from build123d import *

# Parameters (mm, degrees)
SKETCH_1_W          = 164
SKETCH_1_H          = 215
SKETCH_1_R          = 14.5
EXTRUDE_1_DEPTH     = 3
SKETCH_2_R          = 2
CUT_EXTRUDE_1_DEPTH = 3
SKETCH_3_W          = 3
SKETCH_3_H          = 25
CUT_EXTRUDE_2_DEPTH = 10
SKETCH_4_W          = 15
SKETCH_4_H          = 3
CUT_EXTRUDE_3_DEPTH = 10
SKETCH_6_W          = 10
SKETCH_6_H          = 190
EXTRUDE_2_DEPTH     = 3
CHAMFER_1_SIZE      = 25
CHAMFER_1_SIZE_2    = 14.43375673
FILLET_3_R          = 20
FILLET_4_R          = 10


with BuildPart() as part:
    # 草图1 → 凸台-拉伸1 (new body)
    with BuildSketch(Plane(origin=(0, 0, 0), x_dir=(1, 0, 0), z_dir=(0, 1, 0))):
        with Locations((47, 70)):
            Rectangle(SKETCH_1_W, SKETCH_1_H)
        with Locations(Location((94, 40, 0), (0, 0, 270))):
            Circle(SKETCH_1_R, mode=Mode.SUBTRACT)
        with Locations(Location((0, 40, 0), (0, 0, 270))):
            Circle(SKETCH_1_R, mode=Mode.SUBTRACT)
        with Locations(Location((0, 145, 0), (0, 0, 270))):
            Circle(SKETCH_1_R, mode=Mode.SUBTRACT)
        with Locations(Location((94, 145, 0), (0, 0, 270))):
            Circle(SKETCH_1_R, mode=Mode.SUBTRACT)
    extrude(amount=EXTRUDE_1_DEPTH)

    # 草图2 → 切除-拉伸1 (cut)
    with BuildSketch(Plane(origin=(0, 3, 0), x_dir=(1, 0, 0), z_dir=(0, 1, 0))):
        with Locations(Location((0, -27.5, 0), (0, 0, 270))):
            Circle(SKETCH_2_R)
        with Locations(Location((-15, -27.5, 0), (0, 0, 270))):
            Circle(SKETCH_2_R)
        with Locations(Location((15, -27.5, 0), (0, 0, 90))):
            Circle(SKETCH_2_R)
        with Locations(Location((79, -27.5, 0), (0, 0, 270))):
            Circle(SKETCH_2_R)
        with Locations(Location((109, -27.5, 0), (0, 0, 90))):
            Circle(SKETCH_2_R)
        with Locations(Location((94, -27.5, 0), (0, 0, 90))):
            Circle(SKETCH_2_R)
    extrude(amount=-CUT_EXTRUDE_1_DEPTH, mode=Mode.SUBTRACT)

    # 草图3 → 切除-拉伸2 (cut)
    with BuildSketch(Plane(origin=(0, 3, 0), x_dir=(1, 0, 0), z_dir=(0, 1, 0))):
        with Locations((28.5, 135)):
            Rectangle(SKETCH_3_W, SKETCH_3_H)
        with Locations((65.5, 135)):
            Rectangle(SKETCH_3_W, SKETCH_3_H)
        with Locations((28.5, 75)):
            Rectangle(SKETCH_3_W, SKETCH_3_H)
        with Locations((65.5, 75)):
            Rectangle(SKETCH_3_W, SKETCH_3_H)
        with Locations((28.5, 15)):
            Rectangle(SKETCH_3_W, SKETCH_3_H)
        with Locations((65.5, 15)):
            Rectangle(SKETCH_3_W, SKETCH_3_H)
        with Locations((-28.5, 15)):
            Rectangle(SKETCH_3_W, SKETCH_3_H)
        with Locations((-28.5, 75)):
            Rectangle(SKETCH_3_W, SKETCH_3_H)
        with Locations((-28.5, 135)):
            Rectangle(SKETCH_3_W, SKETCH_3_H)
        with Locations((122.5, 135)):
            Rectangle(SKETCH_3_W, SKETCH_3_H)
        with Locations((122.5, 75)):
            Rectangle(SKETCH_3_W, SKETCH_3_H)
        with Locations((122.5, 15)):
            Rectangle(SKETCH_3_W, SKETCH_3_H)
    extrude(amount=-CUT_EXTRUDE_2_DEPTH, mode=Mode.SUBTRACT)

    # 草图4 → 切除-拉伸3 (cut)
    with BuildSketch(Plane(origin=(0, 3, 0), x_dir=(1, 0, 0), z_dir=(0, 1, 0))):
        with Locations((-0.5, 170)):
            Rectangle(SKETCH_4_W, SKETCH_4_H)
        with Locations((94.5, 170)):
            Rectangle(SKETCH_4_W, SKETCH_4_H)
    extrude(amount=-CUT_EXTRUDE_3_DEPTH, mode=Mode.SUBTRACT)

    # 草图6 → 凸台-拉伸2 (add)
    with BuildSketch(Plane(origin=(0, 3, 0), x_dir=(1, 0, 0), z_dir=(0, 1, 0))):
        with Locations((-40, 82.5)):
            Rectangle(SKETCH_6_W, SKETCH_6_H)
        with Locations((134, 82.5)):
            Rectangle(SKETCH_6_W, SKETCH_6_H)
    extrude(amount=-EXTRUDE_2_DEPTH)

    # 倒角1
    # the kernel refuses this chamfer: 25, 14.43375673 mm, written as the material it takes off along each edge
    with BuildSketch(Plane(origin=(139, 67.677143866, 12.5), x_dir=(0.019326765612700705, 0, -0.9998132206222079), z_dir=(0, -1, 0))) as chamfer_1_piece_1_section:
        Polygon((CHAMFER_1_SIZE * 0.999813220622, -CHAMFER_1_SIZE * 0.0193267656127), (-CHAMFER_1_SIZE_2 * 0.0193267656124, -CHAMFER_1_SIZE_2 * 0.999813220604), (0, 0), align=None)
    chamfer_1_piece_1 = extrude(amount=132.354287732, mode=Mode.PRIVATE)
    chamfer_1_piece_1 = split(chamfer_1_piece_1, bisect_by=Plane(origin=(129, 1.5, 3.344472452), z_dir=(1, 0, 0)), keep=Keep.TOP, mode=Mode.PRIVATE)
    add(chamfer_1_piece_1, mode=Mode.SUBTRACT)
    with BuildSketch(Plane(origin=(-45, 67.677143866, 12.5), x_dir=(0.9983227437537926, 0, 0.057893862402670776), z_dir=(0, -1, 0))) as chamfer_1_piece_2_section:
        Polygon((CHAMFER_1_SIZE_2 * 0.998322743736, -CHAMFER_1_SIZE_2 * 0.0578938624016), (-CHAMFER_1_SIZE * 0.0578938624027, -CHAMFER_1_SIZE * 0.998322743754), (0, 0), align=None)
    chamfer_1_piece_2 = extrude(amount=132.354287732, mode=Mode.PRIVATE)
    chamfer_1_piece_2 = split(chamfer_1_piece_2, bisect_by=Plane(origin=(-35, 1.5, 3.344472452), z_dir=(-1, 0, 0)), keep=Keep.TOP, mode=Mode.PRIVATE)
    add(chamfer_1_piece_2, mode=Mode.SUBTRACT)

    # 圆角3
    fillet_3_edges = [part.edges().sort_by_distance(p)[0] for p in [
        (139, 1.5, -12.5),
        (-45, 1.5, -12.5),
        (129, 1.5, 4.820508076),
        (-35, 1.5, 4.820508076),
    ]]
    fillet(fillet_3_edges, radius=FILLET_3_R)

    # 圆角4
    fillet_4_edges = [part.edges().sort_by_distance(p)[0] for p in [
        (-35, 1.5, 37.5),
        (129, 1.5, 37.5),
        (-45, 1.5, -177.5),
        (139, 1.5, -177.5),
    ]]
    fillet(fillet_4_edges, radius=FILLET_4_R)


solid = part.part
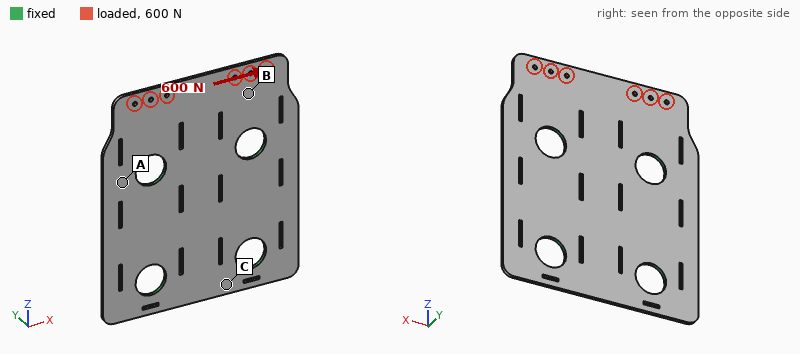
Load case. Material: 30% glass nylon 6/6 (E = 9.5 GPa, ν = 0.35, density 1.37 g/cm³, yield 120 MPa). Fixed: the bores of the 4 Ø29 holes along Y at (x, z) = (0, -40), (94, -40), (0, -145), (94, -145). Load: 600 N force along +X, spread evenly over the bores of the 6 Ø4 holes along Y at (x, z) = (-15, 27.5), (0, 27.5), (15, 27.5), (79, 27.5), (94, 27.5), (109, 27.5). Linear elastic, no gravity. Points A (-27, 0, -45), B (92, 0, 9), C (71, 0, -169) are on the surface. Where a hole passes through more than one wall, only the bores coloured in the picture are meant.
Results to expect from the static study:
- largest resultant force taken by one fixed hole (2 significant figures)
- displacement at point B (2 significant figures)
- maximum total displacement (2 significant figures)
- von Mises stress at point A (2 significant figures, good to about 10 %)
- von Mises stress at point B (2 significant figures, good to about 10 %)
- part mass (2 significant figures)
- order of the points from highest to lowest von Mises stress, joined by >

390 N
24 µm
43 µm
1.2 MPa
2.1 MPa
140 g
B > A > C
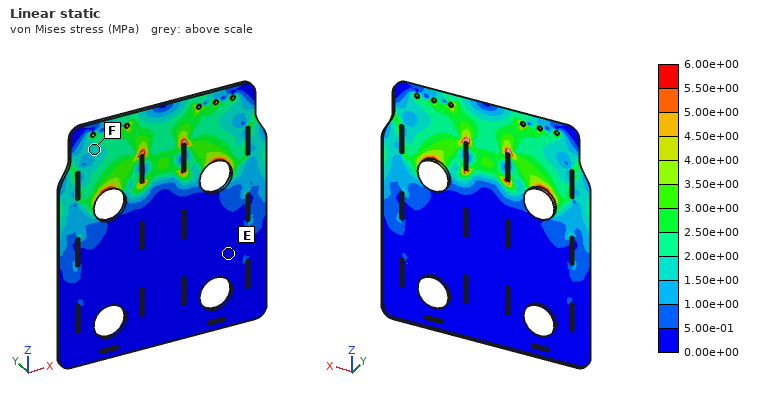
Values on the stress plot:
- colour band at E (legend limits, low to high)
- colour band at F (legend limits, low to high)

0.00e+00 to 5.00e-01 MPa
1.50e+00 to 2.00e+00 MPa
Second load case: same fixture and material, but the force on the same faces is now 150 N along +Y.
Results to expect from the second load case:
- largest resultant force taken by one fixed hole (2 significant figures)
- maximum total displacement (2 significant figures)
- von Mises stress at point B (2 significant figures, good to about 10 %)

76 N
3.2 mm
10.0 MPa
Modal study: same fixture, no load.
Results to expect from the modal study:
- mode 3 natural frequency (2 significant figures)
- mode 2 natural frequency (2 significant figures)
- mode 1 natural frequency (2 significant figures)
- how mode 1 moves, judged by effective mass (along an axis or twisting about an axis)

610 Hz
410 Hz
290 Hz
along Y
